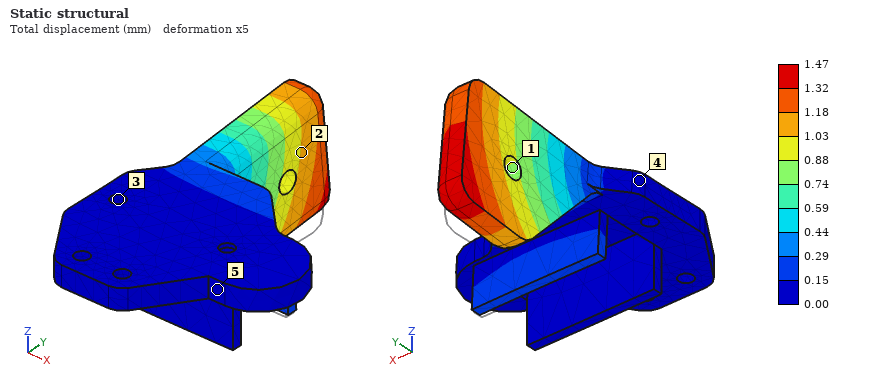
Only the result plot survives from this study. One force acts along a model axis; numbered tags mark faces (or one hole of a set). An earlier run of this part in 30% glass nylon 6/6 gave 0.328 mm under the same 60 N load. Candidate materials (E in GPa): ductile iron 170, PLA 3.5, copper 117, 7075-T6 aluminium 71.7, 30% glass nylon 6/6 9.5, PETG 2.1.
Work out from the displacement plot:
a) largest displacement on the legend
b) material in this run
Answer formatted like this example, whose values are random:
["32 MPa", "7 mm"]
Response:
["1.47 mm", "PETG"]
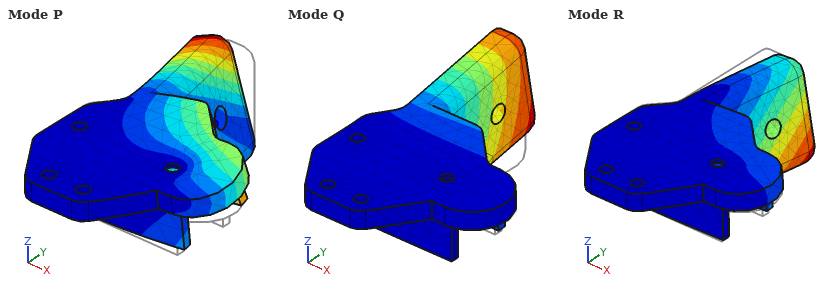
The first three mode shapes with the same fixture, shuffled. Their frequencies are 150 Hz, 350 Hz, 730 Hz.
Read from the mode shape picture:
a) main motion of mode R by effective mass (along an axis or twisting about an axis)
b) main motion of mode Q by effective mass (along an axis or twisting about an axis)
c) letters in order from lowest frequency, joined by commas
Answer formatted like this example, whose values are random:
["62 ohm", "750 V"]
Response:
["along X", "along Z", "Q, R, P"]
